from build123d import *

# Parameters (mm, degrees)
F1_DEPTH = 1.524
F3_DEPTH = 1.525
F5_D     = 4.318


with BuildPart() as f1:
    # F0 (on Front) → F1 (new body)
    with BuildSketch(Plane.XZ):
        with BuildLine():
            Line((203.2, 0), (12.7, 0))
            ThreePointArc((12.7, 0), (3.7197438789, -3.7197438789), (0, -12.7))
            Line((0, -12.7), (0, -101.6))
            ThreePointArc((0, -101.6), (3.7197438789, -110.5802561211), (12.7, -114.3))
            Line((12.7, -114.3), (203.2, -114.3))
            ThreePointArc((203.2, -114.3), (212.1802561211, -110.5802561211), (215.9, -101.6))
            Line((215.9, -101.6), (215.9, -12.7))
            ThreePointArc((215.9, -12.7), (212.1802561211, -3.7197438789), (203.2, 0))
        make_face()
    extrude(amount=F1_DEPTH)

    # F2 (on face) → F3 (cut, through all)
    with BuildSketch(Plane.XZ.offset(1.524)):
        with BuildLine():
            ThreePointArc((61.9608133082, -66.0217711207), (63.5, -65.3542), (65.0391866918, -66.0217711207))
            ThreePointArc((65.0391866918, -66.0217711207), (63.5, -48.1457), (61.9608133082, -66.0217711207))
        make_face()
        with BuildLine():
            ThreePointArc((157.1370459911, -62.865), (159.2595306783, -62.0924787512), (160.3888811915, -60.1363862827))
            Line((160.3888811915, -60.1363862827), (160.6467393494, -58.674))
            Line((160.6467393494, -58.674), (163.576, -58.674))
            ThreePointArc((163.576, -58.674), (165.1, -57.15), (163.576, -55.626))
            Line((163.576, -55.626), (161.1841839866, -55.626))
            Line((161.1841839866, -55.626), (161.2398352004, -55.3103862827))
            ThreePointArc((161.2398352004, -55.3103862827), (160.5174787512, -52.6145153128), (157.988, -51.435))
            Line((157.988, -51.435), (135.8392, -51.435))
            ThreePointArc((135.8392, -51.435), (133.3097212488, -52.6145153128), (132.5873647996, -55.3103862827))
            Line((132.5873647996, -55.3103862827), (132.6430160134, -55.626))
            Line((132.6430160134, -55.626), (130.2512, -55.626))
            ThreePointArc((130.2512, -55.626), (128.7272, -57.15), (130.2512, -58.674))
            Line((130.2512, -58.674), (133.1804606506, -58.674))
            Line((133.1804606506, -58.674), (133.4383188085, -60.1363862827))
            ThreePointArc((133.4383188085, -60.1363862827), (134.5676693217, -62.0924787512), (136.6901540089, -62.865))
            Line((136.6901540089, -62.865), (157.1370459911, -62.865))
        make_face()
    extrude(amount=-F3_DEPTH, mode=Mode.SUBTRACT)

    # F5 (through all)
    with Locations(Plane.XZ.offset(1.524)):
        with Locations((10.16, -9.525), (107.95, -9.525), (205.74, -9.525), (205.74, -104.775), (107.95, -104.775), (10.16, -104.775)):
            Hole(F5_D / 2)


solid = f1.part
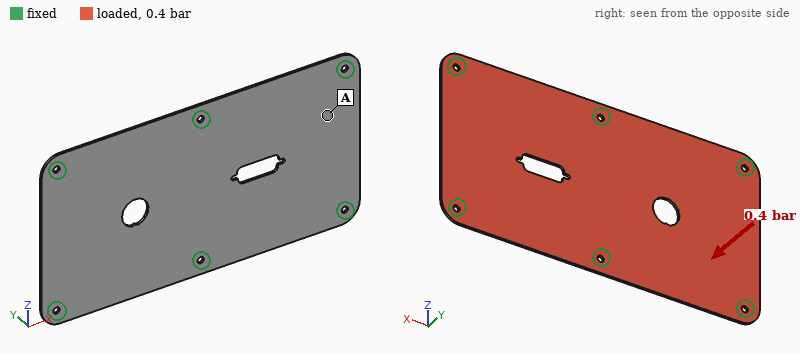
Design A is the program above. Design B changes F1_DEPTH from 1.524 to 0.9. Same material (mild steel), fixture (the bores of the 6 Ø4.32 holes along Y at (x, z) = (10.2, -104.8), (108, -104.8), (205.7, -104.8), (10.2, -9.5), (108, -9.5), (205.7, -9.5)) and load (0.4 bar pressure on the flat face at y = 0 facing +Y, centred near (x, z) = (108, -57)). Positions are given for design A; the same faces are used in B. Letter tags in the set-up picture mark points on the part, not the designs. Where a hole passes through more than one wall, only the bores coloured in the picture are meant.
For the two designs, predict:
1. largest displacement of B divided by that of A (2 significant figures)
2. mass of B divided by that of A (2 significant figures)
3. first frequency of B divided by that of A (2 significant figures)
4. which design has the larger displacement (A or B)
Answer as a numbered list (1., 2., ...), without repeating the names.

1. 4.8
2. 0.59
3. 0.60
4. B
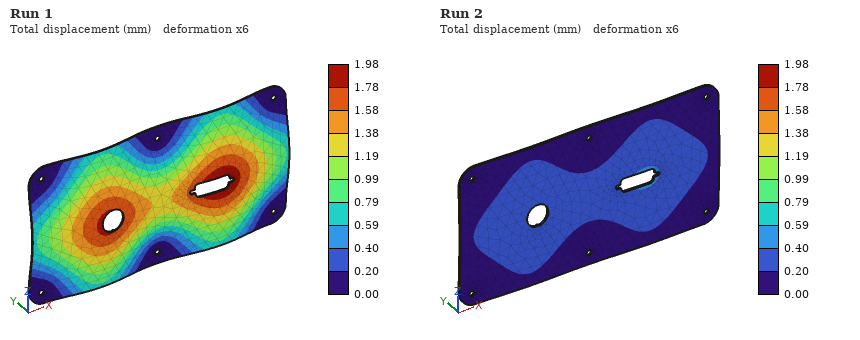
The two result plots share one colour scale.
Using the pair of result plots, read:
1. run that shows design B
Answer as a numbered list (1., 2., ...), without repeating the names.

1. Run 1
